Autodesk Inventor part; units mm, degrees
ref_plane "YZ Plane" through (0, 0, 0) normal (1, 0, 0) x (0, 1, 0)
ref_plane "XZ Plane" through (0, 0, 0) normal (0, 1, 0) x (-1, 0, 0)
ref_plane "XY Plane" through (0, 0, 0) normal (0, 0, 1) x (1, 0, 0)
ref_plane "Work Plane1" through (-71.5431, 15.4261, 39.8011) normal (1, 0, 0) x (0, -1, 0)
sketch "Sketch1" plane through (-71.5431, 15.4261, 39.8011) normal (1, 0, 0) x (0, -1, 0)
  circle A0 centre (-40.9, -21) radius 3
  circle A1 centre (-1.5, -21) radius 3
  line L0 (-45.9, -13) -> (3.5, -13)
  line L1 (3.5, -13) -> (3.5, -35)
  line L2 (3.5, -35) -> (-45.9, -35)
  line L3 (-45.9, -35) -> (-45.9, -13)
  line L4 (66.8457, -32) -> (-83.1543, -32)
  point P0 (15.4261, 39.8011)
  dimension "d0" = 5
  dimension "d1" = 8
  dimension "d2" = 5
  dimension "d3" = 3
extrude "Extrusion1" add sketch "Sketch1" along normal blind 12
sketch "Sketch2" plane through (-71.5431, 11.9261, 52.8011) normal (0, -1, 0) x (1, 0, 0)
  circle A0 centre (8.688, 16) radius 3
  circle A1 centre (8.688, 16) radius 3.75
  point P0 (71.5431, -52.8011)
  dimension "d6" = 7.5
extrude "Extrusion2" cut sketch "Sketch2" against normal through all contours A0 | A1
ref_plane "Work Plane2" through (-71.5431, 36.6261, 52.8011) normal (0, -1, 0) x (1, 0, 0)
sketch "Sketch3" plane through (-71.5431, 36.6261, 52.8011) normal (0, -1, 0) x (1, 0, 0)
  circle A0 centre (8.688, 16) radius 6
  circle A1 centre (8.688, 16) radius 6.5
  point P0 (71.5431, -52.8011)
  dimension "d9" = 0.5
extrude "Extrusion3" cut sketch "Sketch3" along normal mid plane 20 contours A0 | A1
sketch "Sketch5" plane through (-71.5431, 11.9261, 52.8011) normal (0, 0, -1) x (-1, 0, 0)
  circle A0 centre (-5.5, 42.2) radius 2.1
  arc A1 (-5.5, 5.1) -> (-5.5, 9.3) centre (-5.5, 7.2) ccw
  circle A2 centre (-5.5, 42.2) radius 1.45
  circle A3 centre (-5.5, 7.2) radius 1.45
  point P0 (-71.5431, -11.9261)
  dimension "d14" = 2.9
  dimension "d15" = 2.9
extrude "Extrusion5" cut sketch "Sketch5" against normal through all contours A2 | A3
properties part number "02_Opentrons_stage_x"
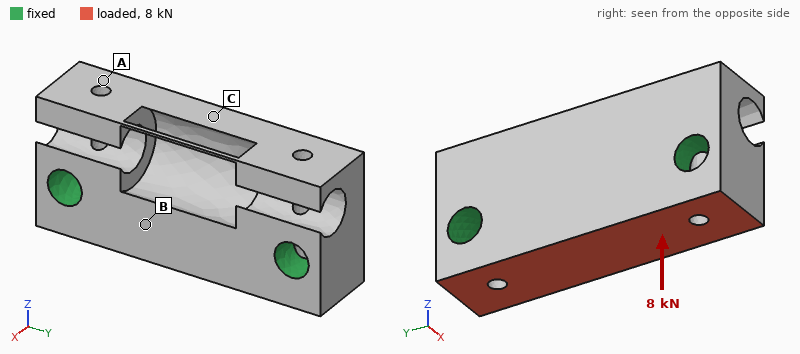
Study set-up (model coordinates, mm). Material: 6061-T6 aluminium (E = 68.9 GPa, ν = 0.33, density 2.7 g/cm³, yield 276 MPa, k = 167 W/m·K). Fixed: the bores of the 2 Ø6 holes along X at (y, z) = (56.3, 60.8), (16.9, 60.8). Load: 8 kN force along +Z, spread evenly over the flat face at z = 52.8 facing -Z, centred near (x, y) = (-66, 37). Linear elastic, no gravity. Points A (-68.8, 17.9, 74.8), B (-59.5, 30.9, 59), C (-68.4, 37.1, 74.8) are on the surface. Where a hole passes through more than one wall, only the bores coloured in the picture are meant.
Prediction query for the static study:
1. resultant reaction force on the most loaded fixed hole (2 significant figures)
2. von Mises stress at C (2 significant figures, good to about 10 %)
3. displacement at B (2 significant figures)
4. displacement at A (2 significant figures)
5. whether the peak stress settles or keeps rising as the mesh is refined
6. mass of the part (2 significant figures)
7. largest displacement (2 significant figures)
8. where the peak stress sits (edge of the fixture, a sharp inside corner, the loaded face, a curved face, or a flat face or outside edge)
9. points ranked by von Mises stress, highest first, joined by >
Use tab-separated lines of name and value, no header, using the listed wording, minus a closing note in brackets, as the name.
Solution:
resultant reaction force on the most loaded fixed hole	4.1 kN
von Mises stress at C	34 MPa
displacement at B	14 µm
displacement at A	5.5 µm
whether the peak stress settles or keeps rising as the mesh is refined	keeps rising
mass of the part	24 g
largest displacement	17 µm
where the peak stress sits	edge of the fixture
points ranked by von Mises stress, highest first, joined by >	C > B > A
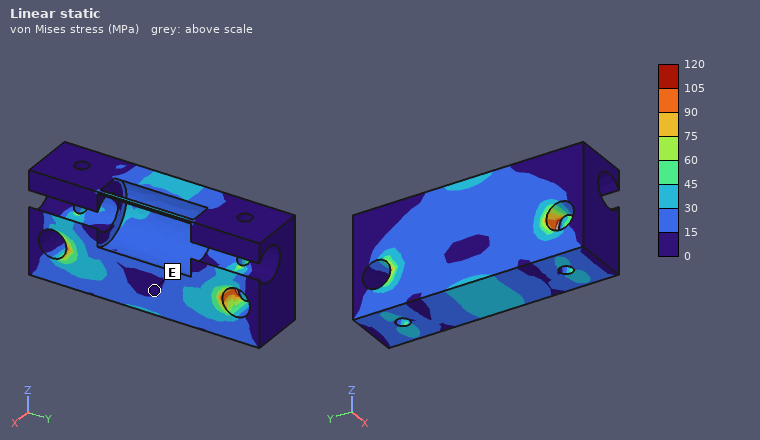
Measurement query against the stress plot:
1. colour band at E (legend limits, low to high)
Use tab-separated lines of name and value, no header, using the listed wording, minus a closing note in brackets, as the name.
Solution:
colour band at E	0 to 15 MPa
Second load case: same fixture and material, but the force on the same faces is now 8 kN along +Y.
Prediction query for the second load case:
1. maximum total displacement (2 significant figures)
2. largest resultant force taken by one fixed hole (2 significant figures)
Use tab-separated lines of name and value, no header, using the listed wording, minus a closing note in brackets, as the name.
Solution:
maximum total displacement	8.0 µm
largest resultant force taken by one fixed hole	4.2 kN
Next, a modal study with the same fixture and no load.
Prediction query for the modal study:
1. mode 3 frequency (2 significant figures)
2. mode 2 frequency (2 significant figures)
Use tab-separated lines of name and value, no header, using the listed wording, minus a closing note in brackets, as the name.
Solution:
mode 3 frequency	10 kHz
mode 2 frequency	8600 Hz
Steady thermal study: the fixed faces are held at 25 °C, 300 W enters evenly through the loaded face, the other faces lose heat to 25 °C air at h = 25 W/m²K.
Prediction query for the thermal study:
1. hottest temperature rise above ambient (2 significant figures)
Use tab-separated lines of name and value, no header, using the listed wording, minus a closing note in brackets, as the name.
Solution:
hottest temperature rise above ambient	58 K
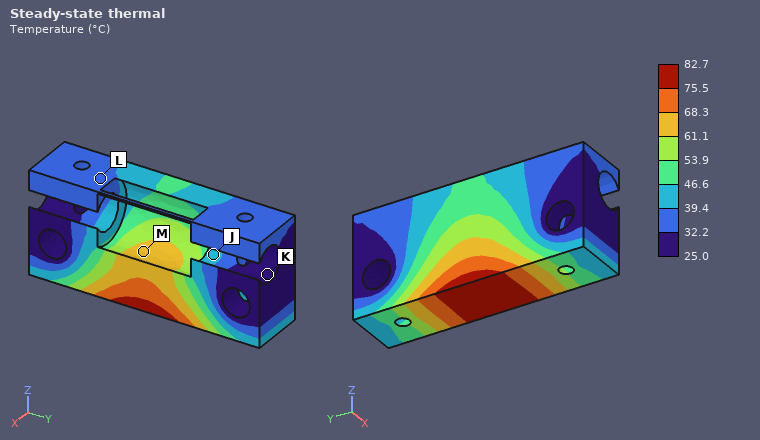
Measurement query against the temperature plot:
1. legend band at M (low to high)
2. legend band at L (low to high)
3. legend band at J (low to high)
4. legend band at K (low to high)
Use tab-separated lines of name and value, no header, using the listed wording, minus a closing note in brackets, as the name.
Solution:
legend band at M	61.1 to 68.3 °C
legend band at L	32.2 to 39.4 °C
legend band at J	39.4 to 46.6 °C
legend band at K	25.0 to 32.2 °C
